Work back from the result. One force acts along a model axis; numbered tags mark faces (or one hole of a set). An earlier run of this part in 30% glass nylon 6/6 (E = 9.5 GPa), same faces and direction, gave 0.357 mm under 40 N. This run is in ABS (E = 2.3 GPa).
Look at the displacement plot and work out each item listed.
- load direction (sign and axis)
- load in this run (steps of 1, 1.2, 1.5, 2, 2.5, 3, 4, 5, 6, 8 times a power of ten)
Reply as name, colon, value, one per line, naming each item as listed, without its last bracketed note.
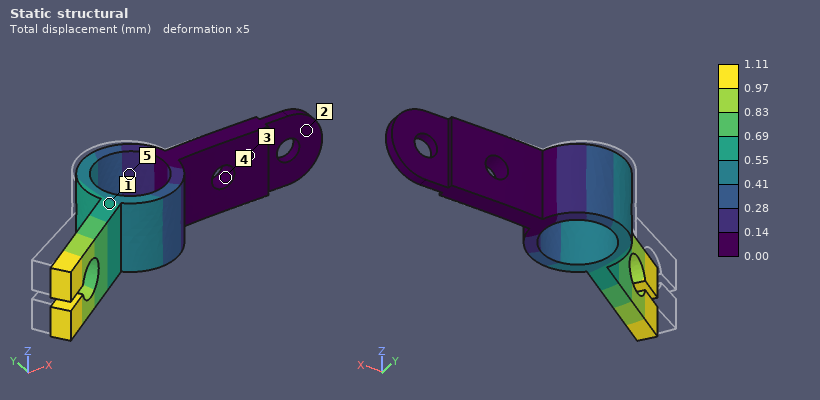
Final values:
load direction: -Y
load in this run: 30 N
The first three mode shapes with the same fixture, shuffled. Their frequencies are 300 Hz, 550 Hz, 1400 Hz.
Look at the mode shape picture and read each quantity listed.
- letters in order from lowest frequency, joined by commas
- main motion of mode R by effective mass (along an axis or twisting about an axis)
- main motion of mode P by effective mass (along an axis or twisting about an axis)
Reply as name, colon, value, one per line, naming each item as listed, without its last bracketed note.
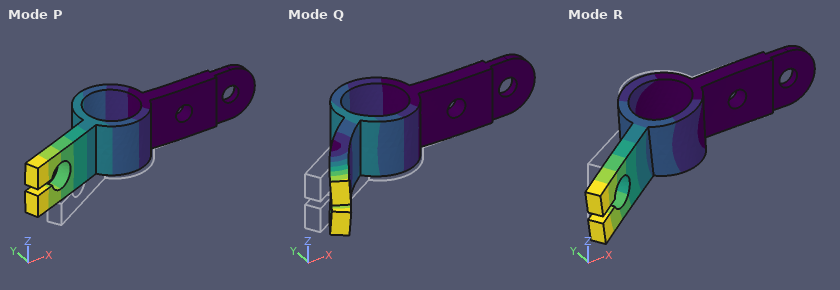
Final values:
letters in order from lowest frequency, joined by commas: P, R, Q
main motion of mode R by effective mass: along Z
main motion of mode P by effective mass: along Y
